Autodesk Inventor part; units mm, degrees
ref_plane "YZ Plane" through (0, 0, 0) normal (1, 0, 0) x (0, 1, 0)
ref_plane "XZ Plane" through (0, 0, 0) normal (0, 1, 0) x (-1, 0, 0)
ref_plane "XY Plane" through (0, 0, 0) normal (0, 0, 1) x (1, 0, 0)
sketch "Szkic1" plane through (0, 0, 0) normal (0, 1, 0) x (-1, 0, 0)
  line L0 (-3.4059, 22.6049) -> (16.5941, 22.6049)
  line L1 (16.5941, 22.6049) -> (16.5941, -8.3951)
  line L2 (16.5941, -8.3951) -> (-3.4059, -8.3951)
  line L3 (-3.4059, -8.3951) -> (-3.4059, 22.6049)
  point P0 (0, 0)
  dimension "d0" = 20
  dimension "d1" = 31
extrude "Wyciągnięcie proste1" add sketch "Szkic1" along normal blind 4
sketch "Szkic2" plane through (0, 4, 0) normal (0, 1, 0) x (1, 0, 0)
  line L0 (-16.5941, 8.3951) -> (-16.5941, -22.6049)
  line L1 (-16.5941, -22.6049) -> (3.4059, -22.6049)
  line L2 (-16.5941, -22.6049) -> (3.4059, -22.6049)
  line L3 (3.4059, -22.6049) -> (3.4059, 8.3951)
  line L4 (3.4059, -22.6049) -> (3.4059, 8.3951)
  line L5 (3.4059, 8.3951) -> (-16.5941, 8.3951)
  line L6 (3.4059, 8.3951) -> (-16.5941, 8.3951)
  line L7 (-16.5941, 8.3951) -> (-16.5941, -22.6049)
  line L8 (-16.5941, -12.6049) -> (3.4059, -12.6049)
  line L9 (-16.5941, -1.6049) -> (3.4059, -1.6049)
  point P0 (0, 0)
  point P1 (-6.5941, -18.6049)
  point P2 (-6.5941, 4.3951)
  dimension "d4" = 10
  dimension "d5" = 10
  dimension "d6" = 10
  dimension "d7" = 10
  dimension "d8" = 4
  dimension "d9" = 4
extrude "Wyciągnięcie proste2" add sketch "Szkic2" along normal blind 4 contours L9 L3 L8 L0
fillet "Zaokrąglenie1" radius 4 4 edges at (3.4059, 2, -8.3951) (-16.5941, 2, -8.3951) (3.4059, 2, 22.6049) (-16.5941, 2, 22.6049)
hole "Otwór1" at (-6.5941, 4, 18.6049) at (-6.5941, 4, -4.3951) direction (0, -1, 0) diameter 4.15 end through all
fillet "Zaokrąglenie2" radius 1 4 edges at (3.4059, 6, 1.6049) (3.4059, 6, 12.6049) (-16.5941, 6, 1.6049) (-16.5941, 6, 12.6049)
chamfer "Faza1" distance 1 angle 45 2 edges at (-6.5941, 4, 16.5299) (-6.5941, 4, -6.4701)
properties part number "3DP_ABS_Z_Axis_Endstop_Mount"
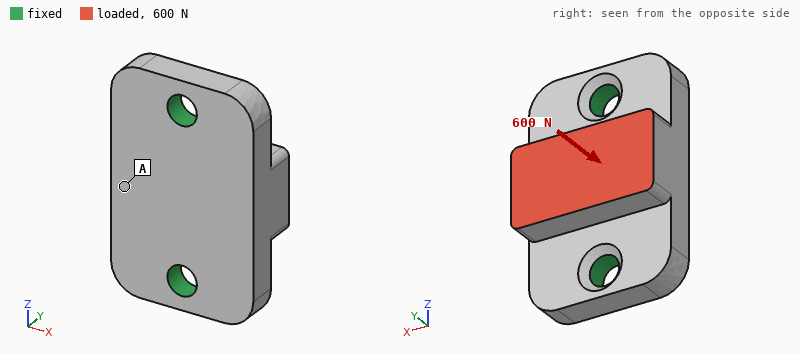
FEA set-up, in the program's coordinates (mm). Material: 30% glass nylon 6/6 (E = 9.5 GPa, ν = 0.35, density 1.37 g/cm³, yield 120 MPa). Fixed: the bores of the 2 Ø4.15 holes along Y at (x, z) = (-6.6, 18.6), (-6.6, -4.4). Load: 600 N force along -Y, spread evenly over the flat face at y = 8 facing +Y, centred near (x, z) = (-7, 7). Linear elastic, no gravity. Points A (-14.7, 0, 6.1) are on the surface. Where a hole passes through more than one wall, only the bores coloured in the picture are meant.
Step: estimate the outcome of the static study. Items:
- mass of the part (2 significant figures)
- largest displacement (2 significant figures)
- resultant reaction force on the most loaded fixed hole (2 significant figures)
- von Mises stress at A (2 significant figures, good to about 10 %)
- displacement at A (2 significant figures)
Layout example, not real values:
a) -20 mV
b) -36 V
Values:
a) 4.4 g
b) 36 µm
c) 340 N
d) 6.2 MPa
e) 34 µm
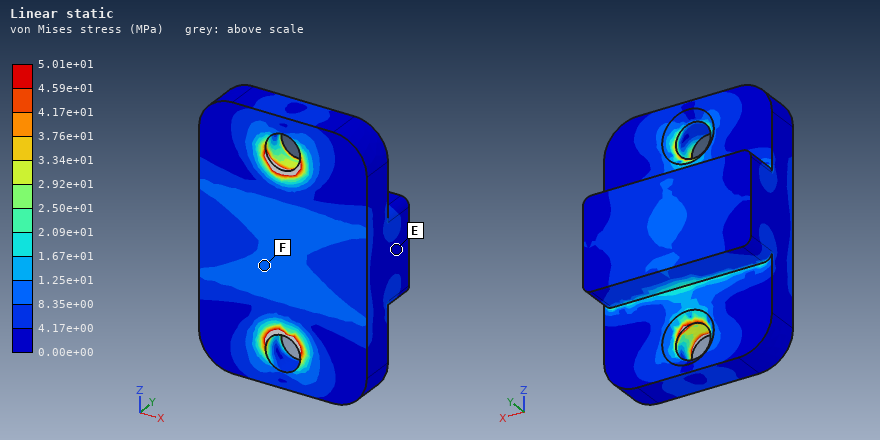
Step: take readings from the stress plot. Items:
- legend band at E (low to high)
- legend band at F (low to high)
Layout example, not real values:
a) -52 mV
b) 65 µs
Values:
a) 0.00e+00 to 4.17e+00 MPa
b) 8.35e+00 to 1.25e+01 MPa
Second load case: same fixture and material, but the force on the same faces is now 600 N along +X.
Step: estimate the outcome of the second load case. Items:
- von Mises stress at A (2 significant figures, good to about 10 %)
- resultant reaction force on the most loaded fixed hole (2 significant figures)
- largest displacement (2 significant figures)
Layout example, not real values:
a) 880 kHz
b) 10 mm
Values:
a) 16 MPa
b) 300 N
c) 0.13 mm
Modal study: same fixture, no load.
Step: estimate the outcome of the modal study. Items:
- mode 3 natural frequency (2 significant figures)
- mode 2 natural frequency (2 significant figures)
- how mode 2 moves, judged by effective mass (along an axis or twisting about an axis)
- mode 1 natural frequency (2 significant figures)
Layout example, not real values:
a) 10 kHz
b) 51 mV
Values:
a) 21 kHz
b) 13 kHz
c) along Y
d) 8400 Hz
